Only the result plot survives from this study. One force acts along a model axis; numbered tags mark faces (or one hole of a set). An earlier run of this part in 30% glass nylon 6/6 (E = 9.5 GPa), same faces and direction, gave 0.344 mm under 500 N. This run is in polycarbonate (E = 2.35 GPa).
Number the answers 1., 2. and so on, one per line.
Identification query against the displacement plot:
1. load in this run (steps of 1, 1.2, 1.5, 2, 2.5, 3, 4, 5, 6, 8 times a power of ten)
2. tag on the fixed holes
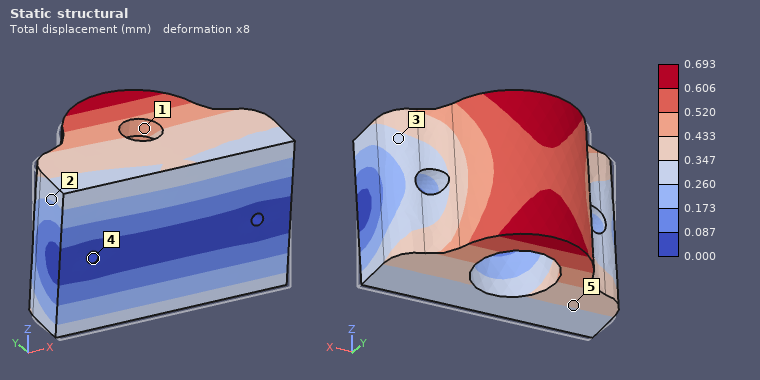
1. 250 N
2. 4
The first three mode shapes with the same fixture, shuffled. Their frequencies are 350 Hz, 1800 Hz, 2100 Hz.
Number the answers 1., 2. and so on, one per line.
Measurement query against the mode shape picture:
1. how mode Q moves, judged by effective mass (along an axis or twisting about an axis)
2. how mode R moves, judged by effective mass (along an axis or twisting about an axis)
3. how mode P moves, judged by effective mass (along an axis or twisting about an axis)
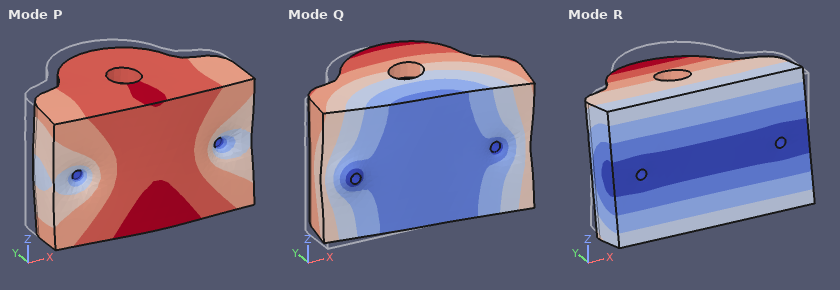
1. along X
2. along Z
3. along Y
